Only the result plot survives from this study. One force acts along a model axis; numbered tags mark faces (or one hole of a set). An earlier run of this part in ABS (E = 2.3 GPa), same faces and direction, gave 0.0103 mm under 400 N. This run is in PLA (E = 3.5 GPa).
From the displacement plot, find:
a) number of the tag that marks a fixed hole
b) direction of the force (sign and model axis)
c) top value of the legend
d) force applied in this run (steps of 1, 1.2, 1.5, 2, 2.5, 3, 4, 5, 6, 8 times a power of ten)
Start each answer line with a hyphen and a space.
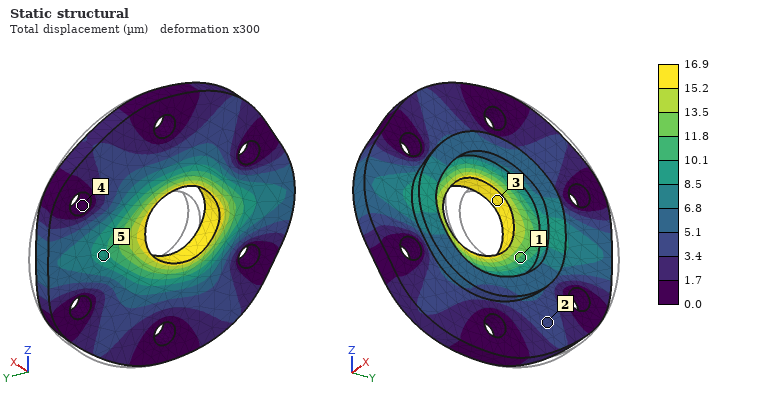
- 4
- -Y
- 16.9 µm
- 1 kN
